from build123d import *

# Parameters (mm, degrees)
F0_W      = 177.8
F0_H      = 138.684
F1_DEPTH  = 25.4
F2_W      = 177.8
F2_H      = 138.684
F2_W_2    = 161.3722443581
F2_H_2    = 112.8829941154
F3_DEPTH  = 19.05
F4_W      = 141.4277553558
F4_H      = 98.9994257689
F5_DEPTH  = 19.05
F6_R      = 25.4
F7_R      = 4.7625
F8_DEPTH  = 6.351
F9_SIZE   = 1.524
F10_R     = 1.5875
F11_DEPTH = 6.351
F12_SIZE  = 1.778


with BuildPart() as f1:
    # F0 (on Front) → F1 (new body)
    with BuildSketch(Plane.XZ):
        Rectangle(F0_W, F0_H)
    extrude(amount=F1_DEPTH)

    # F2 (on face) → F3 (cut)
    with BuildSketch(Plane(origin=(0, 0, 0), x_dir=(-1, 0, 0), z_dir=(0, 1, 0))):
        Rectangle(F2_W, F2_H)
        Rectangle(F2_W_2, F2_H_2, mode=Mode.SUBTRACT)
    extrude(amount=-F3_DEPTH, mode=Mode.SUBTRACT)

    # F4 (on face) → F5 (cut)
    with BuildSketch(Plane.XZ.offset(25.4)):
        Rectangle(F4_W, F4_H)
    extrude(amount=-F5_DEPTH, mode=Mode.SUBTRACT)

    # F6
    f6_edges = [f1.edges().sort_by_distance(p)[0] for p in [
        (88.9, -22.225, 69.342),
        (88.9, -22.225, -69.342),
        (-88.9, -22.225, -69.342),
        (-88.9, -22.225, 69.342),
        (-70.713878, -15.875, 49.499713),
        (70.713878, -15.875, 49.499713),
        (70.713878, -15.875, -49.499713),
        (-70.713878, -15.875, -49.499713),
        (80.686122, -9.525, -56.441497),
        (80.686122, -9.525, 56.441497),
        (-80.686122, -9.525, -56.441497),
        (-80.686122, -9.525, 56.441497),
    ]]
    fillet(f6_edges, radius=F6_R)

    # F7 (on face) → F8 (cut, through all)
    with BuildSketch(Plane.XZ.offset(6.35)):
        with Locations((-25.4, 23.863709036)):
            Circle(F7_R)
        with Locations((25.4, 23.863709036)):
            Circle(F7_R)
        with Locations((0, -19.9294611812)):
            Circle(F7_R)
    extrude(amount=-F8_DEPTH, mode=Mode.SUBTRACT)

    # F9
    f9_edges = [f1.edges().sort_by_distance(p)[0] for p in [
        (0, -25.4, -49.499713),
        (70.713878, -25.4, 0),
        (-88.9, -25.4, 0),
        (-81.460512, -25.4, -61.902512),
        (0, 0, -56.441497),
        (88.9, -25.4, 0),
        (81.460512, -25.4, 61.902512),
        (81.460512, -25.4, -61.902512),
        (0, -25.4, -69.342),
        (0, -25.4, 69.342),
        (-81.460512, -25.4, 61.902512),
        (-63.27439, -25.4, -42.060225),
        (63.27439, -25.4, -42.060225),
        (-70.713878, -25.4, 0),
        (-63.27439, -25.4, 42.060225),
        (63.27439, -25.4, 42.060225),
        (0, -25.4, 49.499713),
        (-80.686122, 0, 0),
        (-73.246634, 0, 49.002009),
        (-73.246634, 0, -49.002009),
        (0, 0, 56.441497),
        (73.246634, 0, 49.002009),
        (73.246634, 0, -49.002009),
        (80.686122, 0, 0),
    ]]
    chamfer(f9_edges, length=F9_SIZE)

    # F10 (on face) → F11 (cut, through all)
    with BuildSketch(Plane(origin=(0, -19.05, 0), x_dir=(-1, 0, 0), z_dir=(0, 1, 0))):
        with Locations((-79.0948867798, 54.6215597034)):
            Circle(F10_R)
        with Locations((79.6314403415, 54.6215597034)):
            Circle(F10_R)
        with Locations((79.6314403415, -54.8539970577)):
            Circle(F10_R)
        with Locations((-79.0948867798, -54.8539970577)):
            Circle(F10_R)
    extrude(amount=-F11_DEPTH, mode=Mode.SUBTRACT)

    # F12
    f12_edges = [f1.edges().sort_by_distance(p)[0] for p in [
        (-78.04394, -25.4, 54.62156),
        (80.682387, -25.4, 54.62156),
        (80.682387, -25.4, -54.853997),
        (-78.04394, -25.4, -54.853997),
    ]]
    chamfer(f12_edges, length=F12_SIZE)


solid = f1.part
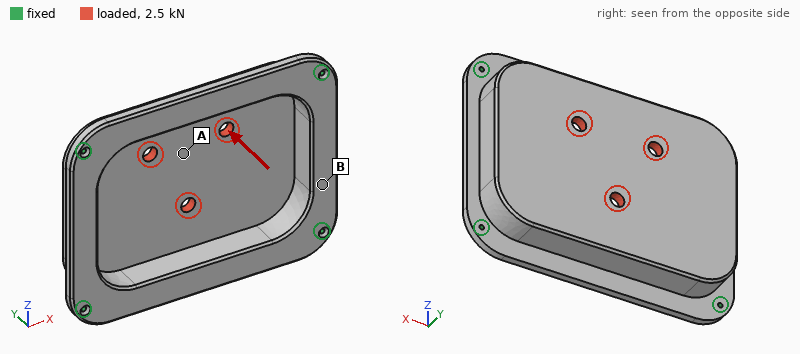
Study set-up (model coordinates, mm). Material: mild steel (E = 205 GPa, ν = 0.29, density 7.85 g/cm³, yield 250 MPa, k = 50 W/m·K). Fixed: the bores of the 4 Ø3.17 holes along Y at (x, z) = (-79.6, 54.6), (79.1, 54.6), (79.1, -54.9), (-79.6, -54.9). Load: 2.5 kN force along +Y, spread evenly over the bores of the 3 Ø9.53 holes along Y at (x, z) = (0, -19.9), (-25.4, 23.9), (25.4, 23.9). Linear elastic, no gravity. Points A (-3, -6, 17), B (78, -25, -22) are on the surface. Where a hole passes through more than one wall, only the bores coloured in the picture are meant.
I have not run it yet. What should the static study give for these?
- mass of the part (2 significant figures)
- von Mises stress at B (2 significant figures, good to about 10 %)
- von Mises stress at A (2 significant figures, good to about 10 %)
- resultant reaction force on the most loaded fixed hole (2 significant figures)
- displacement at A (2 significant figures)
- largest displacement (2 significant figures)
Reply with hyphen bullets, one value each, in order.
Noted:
- 1.8 kg
- 3.9 MPa
- 15 MPa
- 1.3 kN
- 33 µm
- 35 µm
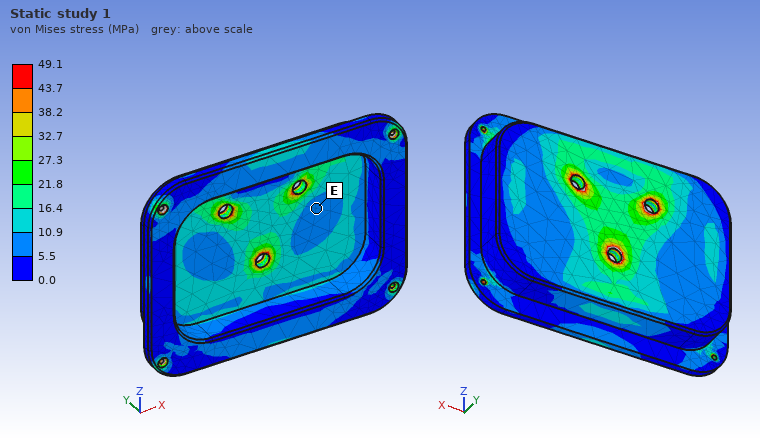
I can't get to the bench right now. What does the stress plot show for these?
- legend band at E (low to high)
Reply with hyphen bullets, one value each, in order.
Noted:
- 5.5 to 10.9 MPa
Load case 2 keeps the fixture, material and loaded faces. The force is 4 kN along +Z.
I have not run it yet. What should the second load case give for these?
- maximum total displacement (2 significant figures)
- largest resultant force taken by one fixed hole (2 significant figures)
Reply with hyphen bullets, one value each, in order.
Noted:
- 5.6 µm
- 1.1 kN
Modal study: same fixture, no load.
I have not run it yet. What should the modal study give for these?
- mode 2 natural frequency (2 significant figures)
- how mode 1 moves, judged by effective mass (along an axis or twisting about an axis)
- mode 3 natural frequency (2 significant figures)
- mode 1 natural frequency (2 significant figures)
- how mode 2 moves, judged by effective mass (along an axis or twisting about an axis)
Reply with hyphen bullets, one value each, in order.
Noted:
- 2700 Hz
- along Y
- 3300 Hz
- 2300 Hz
- twisting about X
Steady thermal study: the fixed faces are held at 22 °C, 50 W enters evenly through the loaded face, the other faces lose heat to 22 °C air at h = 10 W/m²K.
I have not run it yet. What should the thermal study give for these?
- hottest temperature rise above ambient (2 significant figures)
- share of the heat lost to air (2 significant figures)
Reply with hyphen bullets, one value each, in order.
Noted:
- 52 K
- 34 %
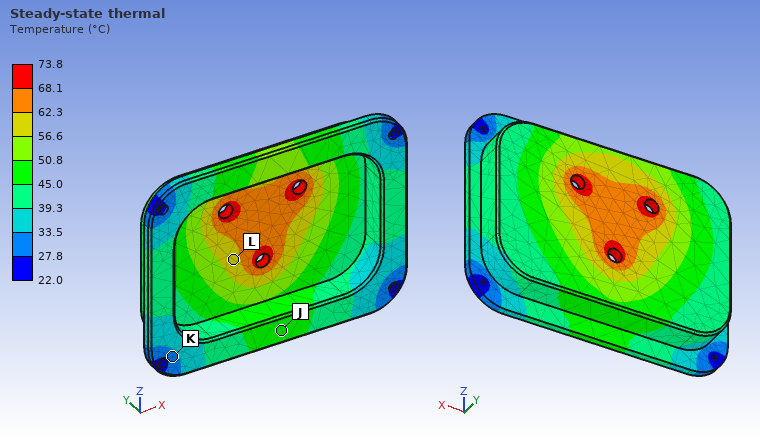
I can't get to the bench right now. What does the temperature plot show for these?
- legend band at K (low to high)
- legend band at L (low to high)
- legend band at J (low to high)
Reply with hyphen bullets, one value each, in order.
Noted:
- 27.8 to 33.5 °C
- 56.6 to 62.3 °C
- 45.0 to 50.8 °C
